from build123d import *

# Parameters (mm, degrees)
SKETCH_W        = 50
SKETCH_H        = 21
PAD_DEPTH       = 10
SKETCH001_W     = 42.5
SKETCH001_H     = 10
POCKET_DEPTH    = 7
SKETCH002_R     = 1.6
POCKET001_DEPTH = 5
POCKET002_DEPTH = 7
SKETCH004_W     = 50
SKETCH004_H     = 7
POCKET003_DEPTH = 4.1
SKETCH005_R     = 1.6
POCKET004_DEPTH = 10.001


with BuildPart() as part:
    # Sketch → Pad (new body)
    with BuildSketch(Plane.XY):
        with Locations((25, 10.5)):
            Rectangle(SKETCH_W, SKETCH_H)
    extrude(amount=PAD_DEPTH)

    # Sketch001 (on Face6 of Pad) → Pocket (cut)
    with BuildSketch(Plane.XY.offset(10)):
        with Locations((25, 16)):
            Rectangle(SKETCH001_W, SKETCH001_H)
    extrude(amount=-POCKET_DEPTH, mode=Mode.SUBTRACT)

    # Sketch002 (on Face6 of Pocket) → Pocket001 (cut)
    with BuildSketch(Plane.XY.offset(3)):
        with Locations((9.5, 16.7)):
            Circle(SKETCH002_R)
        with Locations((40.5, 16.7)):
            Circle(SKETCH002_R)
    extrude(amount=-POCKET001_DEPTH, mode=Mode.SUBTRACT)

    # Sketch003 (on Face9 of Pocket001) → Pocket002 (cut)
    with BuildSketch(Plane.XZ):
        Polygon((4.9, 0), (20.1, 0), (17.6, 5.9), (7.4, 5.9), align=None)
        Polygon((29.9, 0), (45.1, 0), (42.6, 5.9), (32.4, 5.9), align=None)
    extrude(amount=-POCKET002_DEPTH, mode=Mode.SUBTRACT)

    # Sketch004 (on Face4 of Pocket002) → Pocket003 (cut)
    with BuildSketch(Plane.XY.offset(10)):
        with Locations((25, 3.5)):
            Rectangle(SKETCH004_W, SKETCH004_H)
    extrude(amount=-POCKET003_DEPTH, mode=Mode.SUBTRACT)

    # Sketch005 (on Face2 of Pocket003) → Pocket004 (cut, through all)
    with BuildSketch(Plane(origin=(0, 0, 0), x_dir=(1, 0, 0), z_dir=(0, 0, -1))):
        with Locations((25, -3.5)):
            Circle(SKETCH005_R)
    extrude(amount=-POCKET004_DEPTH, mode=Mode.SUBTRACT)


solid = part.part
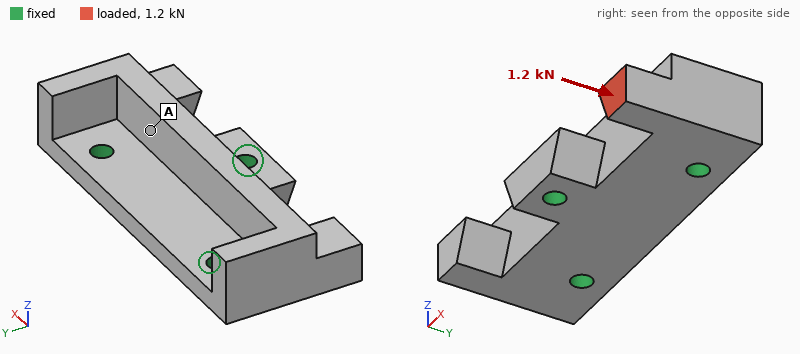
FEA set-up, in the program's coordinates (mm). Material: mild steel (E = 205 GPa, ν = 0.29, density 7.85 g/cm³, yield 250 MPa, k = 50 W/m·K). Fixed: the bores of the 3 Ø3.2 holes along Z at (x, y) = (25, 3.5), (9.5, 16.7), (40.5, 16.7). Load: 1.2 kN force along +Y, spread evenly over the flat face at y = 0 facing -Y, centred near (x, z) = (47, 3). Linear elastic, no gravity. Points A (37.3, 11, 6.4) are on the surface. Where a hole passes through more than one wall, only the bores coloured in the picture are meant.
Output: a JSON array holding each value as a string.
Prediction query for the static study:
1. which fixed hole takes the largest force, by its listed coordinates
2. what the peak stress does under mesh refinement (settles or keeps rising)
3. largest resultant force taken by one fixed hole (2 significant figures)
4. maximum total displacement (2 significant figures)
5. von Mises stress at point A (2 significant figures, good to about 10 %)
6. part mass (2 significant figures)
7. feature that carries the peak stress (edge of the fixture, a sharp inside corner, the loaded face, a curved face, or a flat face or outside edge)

["(40.5, 16.7)", "keeps rising", "1.4 kN", "17 µm", "23 MPa", "39 g", "edge of the fixture"]
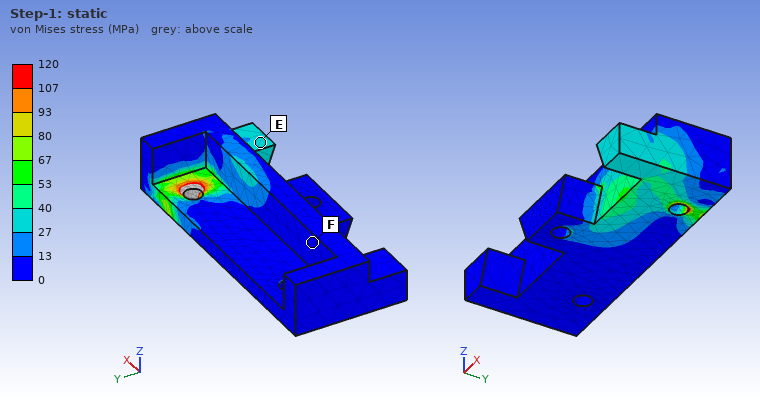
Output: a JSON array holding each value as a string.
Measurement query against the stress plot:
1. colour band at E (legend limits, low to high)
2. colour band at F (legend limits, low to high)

["27 to 40 MPa", "0 to 13 MPa"]
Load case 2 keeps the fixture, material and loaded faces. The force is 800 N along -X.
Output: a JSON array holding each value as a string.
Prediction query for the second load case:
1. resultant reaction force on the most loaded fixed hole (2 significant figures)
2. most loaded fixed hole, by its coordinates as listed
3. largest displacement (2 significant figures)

["550 N", "(25, 3.5)", "26 µm"]
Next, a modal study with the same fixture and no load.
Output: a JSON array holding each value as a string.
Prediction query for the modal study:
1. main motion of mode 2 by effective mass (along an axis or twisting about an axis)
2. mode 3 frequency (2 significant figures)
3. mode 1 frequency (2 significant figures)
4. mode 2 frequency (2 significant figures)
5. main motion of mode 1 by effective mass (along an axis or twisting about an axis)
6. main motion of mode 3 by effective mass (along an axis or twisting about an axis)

["along Z", "22 kHz", "10 kHz", "11 kHz", "twisting about Y", "along X"]
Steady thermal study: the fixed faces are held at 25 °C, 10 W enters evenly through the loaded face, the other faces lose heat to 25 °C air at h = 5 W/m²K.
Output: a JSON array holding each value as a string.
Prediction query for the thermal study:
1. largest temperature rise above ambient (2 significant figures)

["79 K"]
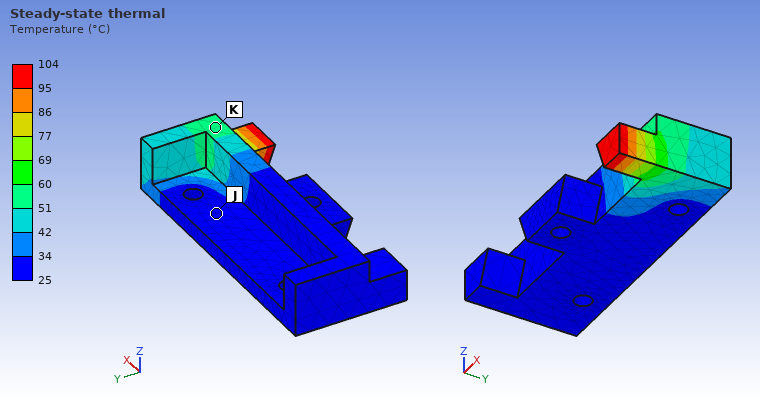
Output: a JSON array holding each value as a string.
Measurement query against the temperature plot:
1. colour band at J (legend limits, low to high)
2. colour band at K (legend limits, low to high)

["25 to 34 °C", "51 to 60 °C"]
